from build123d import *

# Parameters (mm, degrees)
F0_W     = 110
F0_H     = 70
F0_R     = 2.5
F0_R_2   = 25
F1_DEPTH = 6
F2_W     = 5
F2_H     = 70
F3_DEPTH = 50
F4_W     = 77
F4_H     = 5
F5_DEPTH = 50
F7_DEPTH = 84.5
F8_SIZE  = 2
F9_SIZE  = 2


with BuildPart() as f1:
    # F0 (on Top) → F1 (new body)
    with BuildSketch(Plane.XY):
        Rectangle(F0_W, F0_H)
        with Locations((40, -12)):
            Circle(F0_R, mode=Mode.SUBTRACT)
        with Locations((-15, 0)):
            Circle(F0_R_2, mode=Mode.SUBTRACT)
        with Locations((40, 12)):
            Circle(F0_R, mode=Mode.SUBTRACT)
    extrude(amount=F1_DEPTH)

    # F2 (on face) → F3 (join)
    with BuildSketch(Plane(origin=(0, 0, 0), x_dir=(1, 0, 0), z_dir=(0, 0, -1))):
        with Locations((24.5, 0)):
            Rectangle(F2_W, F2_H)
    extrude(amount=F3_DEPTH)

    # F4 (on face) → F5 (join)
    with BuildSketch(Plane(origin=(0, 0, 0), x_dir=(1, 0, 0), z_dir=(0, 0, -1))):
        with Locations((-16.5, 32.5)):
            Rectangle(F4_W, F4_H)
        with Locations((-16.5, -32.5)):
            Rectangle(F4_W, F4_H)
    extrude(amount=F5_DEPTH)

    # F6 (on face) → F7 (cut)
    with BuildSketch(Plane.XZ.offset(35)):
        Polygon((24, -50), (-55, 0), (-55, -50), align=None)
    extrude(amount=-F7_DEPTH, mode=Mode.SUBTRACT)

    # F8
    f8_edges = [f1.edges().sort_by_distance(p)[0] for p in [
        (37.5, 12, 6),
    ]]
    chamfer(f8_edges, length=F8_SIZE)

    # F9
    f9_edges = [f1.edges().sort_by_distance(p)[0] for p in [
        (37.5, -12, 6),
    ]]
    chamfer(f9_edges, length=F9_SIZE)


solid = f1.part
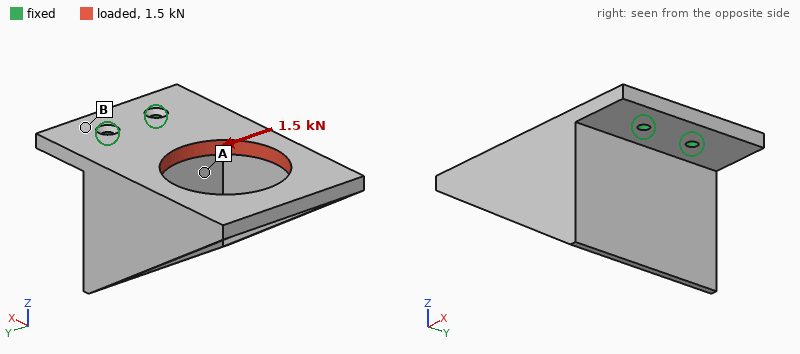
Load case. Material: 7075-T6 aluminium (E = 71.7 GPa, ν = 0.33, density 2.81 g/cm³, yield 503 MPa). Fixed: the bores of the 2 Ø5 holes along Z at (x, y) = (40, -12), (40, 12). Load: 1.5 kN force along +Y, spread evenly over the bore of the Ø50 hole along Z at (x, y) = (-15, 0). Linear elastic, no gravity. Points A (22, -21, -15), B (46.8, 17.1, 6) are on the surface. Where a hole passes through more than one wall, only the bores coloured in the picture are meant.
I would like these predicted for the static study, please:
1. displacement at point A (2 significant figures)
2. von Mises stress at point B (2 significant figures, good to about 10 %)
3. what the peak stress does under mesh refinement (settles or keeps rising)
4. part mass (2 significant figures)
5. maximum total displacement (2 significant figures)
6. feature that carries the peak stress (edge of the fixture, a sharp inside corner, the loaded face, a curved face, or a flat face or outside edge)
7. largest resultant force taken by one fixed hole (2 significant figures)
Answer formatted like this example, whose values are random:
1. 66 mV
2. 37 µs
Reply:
1. 0.017 mm
2. 13 MPa
3. keeps rising
4. 200 g
5. 0.11 mm
6. edge of the fixture
7. 3.1 kN
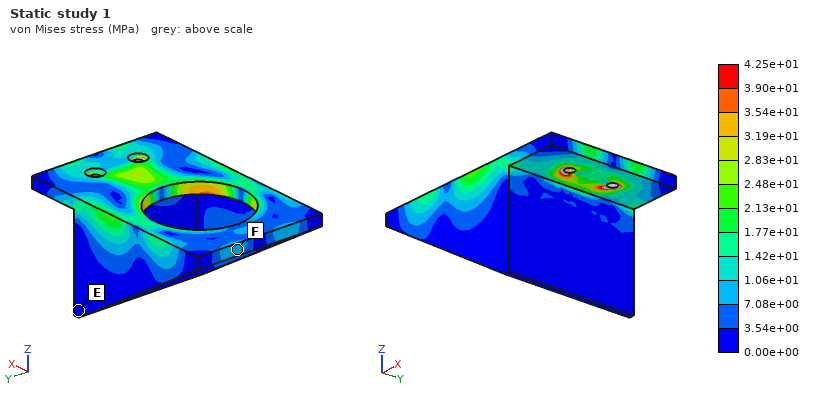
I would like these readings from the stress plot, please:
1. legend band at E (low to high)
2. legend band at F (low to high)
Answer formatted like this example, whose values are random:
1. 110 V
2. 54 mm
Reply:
1. 0.00e+00 to 3.54e+00 MPa
2. 7.08e+00 to 1.06e+01 MPa
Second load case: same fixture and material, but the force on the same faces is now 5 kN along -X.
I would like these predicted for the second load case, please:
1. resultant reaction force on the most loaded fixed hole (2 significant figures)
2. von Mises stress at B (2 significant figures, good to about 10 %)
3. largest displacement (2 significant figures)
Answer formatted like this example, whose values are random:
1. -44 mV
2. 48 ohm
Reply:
1. 2.5 kN
2. 14 MPa
3. 87 µm
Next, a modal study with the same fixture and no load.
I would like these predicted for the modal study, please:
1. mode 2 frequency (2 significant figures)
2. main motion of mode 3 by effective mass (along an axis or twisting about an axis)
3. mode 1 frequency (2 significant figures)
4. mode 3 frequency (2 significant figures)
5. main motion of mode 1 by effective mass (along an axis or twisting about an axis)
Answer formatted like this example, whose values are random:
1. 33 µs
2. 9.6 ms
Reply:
1. 1200 Hz
2. along Y
3. 500 Hz
4. 2100 Hz
5. along Z
